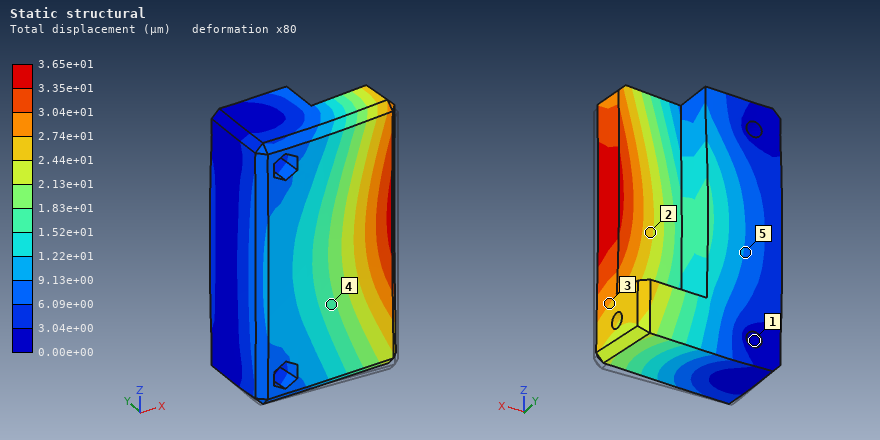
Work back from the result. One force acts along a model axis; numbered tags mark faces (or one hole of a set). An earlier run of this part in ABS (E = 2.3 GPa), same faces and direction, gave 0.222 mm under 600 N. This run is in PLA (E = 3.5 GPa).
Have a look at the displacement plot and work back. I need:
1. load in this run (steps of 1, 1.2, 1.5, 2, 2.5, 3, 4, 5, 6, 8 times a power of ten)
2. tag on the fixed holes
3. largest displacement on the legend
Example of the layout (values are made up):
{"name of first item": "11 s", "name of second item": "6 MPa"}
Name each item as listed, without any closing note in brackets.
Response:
{"load in this run": "150 N", "tag on the fixed holes": "1", "largest displacement on the legend": "3.65e+01 µm"}
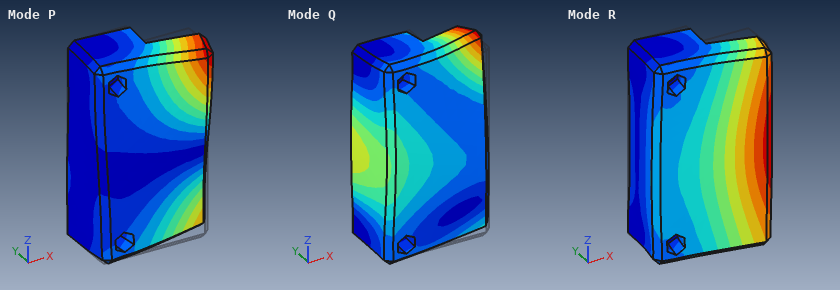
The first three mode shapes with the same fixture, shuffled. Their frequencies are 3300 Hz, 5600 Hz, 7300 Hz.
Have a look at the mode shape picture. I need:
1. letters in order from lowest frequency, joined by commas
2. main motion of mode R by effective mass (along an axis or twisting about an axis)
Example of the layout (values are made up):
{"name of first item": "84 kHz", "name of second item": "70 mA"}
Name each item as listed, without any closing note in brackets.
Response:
{"letters in order from lowest frequency, joined by commas": "R, P, Q", "main motion of mode R by effective mass": "along Y"}
